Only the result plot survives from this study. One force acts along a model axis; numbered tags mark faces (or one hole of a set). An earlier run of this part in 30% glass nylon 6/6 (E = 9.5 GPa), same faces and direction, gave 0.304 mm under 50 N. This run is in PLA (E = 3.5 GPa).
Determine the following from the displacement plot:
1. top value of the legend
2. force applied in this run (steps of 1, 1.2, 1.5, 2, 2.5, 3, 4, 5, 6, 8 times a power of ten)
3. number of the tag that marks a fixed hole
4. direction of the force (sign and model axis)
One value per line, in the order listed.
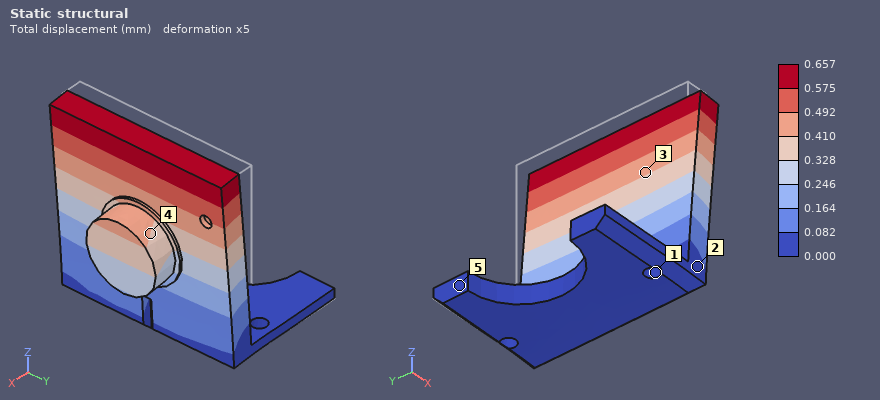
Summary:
0.657 mm
40 N
1
+X
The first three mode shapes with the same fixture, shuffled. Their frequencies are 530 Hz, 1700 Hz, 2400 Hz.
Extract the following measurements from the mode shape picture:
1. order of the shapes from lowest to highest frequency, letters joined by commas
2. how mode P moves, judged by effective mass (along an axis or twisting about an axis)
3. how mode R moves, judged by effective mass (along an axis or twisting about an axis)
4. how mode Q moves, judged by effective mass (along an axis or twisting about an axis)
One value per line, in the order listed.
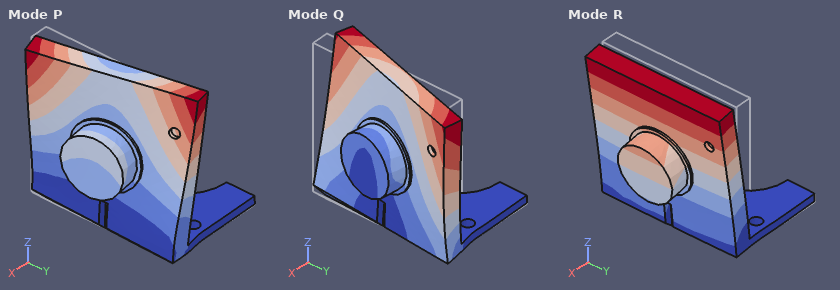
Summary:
R, Q, P
along Y
along X
along Y
